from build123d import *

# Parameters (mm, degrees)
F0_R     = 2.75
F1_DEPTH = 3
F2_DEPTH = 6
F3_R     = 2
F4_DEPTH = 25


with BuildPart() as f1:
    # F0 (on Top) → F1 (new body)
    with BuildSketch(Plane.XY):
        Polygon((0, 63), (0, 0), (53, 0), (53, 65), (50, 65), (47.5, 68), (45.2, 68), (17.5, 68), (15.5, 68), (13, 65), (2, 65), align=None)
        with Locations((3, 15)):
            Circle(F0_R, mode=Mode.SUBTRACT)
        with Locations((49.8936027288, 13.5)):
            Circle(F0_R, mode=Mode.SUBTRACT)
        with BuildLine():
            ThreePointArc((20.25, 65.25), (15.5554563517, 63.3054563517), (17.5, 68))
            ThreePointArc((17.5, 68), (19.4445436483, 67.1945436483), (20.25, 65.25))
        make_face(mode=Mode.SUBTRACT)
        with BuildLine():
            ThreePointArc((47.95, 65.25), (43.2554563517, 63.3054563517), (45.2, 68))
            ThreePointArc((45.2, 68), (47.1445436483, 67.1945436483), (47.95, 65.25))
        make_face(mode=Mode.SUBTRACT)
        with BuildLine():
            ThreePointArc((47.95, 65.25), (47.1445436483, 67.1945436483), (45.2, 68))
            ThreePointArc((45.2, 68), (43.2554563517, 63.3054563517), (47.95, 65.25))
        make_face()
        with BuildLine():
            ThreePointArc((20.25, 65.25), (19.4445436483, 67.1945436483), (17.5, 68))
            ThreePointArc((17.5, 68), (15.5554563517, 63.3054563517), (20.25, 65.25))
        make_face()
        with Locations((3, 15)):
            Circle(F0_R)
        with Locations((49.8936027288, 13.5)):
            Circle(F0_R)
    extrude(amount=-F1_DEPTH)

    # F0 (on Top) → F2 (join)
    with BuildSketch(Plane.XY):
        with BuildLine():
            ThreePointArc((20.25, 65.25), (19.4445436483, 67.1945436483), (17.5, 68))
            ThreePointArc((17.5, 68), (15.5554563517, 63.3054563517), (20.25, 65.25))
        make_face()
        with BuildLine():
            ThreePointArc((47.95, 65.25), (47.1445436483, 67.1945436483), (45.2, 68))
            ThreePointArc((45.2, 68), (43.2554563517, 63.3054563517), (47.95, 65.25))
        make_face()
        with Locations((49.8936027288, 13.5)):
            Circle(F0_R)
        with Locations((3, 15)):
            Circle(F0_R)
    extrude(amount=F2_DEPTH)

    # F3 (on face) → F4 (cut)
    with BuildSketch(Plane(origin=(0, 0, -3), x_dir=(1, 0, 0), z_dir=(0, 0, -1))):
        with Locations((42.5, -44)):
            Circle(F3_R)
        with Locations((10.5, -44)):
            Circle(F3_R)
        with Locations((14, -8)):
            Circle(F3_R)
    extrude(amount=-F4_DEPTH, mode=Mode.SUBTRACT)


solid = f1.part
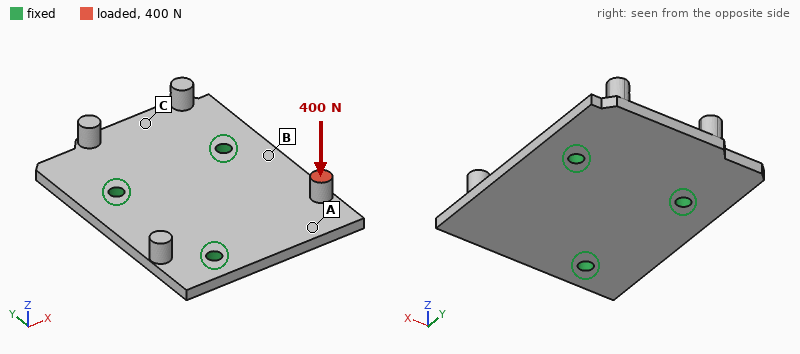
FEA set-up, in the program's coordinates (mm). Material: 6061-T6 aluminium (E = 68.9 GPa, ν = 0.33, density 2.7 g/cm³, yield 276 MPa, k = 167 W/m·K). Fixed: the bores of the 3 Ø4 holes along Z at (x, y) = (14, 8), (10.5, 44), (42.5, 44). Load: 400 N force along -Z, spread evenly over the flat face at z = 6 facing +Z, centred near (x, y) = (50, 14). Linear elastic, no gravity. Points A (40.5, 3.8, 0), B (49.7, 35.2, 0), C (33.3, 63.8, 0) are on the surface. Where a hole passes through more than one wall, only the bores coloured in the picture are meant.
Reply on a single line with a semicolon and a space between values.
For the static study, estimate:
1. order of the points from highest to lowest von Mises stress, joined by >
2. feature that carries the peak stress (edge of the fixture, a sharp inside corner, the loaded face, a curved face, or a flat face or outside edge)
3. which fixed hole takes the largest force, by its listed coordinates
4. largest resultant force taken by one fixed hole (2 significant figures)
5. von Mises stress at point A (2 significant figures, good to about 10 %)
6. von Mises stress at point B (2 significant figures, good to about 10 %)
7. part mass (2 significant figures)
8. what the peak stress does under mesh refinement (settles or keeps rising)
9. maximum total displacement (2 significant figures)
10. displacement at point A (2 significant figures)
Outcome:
B > A > C; edge of the fixture; (42.5, 44); 310 N; 49 MPa; 100 MPa; 30 g; keeps rising; 0.63 mm; 0.34 mm
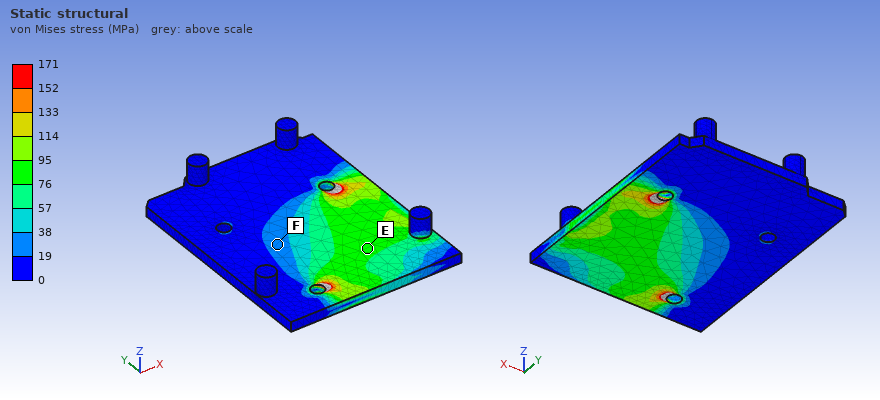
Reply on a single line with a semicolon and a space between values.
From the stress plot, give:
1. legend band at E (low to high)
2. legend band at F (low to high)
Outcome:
76 to 95 MPa; 19 to 38 MPa
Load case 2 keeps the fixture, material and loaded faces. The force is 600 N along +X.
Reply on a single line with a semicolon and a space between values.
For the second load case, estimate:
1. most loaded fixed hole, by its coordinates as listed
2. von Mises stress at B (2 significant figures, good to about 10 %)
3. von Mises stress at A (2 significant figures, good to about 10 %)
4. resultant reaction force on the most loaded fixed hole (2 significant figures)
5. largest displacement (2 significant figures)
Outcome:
(14, 8); 61 MPa; 73 MPa; 420 N; 0.32 mm
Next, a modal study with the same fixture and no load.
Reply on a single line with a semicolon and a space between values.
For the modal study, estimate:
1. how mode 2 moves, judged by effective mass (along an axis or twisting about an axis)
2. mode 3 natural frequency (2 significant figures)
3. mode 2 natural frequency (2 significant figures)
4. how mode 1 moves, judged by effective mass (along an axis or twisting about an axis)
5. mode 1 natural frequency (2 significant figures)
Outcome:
along Z; 6100 Hz; 3800 Hz; along Z; 2700 Hz
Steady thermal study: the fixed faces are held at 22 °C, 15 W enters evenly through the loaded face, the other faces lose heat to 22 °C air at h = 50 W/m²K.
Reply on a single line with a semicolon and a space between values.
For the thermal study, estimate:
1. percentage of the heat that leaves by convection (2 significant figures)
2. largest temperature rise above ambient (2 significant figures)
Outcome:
14 %; 53 K
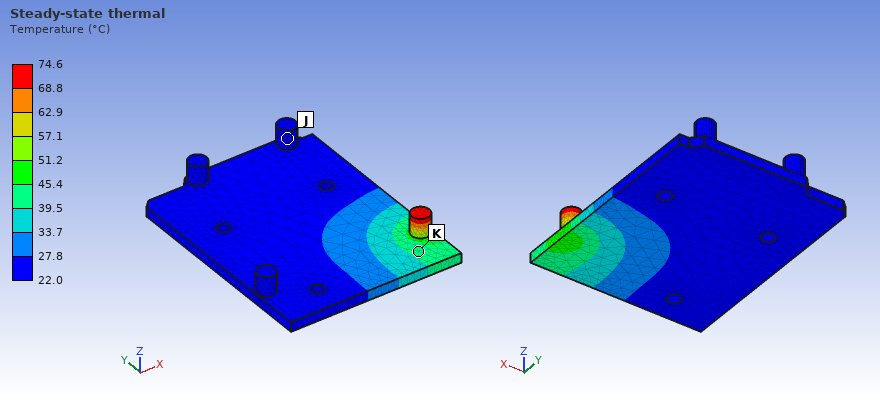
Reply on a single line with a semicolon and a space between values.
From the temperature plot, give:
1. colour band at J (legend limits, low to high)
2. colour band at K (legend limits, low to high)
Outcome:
22.0 to 27.8 °C; 39.5 to 45.4 °C
